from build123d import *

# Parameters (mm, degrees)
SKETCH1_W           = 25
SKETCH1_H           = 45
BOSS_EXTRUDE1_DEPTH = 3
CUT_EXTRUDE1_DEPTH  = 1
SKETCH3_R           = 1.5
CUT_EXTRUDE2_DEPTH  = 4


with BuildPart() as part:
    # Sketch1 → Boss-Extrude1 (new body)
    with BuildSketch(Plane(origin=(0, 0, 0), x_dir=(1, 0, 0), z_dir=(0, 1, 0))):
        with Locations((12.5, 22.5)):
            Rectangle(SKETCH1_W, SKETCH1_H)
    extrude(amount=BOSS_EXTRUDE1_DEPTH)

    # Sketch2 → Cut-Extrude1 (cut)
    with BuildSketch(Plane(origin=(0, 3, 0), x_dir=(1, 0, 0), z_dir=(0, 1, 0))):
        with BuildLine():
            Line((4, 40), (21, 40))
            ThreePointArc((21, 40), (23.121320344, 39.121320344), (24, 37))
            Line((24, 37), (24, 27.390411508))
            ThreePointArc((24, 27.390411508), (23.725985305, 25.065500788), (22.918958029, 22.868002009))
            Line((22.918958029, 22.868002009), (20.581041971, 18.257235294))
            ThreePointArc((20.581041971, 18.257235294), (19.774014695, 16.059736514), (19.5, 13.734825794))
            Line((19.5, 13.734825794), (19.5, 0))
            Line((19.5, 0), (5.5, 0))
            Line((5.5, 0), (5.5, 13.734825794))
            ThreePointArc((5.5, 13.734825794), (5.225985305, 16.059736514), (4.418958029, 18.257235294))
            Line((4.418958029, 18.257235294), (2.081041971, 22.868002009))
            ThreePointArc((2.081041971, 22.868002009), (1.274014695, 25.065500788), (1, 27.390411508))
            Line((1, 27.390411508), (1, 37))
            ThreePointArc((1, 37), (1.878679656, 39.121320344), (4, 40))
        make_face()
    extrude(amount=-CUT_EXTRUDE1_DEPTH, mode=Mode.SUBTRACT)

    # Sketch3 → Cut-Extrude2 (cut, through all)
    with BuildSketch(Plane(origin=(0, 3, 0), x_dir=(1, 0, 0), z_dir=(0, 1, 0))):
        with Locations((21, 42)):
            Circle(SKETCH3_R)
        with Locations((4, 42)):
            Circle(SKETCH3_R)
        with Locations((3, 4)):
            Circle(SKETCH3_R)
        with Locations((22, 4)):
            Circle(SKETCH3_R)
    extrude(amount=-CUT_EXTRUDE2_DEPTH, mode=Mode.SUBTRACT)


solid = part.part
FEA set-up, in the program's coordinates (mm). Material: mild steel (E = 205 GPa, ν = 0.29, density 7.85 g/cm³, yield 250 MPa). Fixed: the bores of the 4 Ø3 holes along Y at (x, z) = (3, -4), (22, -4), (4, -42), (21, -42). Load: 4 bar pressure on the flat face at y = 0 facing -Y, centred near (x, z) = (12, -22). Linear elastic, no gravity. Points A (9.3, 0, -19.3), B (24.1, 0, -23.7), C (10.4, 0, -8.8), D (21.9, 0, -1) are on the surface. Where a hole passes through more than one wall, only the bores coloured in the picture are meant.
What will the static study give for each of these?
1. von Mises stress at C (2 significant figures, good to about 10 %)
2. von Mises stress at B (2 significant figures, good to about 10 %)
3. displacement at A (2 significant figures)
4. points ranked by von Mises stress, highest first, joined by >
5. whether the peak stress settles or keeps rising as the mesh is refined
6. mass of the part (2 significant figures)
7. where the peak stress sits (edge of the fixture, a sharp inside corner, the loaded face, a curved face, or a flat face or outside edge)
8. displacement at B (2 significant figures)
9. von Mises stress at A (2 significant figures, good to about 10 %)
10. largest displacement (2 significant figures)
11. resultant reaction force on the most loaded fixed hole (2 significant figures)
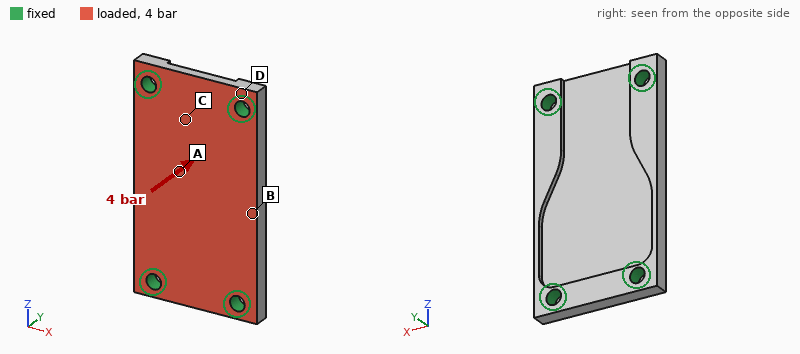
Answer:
13 MPa
28 MPa
8.8 µm
B > A > C > D
keeps rising
20 g
edge of the fixture
8.7 µm
18 MPa
9.8 µm
120 N
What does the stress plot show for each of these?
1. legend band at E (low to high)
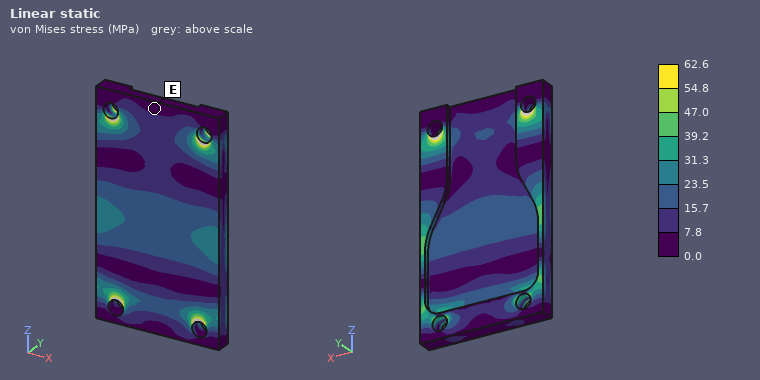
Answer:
0.0 to 7.8 MPa
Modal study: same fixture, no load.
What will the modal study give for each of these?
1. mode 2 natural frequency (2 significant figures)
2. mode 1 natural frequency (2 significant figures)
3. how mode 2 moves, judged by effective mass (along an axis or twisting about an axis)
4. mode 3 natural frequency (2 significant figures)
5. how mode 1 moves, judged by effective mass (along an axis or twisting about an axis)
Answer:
13 kHz
9100 Hz
twisting about Z
23 kHz
along Y
